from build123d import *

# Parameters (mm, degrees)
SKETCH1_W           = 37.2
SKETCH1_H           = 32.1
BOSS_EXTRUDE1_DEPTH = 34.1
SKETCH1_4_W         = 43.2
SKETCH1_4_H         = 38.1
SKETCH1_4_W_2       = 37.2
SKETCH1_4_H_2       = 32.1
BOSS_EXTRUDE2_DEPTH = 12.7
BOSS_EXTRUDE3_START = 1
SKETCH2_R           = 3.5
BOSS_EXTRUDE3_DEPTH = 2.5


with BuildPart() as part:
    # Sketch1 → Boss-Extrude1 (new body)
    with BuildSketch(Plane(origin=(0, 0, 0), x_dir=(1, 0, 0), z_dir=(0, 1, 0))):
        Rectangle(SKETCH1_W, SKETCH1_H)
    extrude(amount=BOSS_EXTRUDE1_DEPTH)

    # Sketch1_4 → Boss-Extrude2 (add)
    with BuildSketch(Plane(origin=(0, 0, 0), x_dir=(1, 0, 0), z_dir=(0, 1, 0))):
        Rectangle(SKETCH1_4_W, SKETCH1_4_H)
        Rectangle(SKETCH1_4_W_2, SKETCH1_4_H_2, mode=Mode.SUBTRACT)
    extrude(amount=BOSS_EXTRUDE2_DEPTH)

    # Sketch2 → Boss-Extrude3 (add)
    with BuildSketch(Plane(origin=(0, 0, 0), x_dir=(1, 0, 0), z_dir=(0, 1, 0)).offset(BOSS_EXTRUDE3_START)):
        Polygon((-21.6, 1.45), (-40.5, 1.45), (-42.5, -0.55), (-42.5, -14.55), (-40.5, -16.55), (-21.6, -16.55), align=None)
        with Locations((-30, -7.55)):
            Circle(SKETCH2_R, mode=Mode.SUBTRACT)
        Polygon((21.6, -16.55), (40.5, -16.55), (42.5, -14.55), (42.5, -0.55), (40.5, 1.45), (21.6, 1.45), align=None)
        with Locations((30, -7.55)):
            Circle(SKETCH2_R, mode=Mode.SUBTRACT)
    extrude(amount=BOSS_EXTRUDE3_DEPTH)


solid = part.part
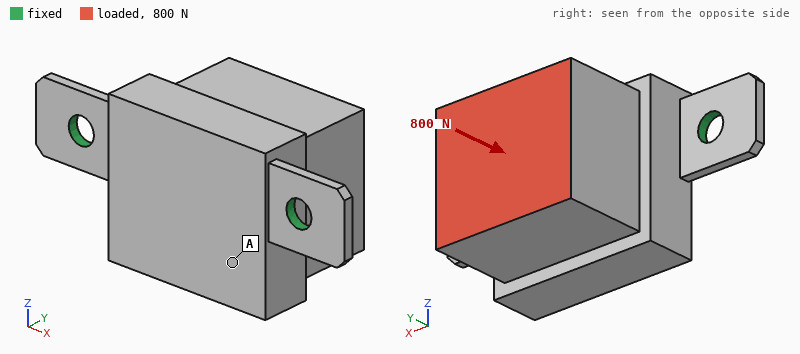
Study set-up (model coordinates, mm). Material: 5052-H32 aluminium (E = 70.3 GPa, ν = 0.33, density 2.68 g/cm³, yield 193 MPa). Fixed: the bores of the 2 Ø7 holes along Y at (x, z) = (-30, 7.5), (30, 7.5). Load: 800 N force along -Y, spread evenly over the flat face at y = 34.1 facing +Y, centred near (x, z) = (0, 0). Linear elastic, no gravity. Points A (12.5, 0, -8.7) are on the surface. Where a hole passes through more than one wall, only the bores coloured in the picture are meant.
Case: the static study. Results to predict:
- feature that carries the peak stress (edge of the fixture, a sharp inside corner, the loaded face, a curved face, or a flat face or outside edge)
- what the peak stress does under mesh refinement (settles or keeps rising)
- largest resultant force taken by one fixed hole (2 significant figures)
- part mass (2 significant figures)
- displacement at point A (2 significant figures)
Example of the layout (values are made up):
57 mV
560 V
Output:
edge of the fixture
keeps rising
430 N
130 g
0.074 mm
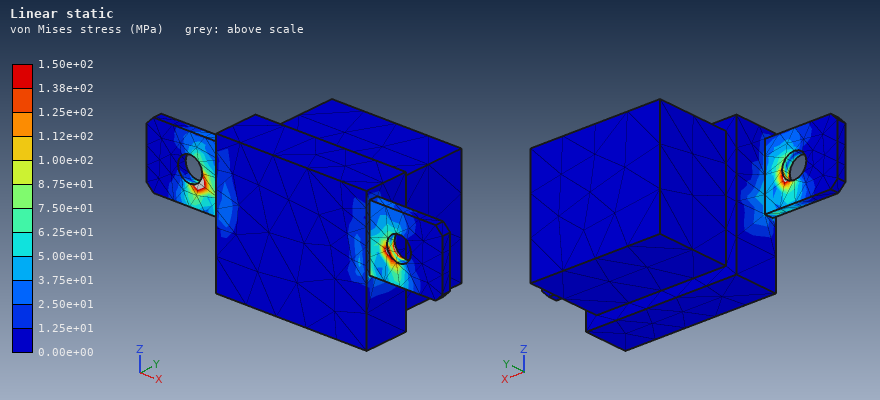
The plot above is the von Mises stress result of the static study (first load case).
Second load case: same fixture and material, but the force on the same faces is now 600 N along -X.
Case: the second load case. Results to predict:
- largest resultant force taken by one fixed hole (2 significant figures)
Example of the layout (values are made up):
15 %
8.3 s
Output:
500 N
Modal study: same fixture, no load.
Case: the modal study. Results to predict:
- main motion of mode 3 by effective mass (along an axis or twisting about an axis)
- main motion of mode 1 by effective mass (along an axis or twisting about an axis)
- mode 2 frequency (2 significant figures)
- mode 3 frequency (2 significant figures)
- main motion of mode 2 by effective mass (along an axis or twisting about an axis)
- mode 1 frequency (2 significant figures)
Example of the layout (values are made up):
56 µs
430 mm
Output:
along X
along Z
4100 Hz
4500 Hz
along Y
840 Hz
